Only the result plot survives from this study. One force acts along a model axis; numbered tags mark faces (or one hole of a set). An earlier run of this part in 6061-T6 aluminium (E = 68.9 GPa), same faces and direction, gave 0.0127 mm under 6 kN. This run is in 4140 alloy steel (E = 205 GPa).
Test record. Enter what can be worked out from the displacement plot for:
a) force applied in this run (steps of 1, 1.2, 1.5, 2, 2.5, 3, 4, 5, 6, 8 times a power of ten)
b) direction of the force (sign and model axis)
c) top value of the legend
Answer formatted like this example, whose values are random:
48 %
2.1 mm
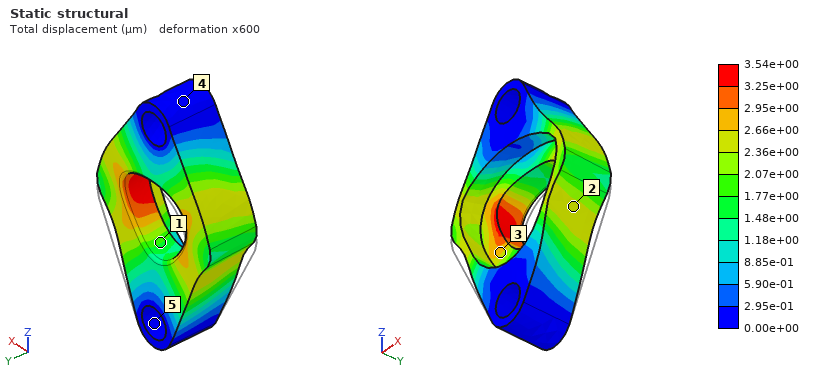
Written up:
5 kN
+Z
3.54e+00 µm
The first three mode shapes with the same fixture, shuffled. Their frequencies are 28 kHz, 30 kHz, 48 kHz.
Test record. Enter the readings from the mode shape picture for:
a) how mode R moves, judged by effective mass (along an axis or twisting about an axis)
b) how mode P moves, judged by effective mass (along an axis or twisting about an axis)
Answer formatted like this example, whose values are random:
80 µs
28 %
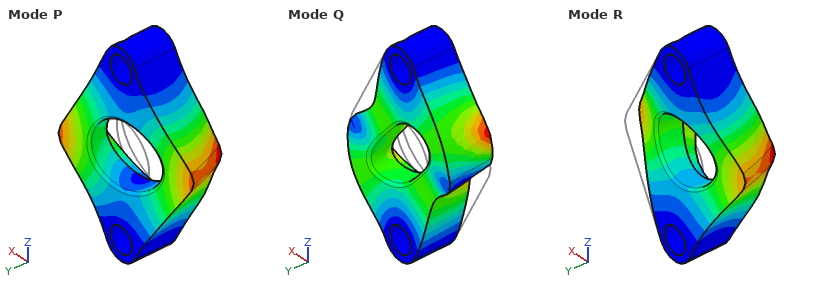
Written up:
along Y
twisting about Z
